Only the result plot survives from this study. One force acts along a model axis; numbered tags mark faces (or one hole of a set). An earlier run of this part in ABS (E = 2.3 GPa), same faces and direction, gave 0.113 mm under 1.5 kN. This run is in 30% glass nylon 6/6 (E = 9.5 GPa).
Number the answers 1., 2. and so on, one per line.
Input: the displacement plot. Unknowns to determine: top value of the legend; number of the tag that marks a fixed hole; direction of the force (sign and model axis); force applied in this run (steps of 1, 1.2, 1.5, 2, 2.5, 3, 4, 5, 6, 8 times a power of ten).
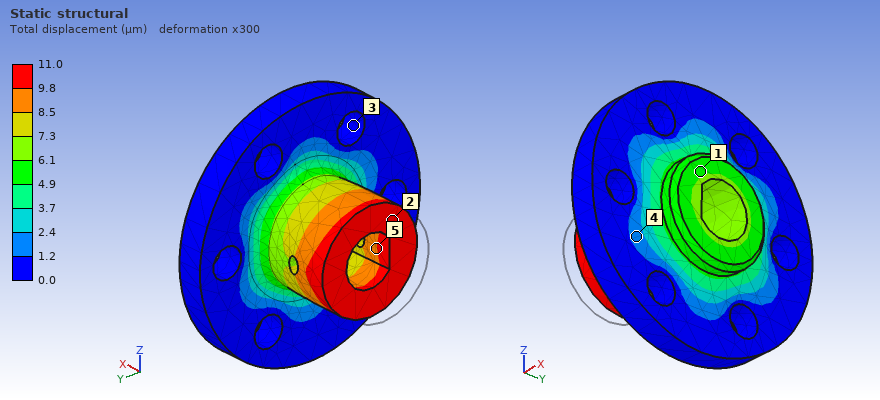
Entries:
1. 11.0 µm
2. 3
3. +X
4. 600 N
